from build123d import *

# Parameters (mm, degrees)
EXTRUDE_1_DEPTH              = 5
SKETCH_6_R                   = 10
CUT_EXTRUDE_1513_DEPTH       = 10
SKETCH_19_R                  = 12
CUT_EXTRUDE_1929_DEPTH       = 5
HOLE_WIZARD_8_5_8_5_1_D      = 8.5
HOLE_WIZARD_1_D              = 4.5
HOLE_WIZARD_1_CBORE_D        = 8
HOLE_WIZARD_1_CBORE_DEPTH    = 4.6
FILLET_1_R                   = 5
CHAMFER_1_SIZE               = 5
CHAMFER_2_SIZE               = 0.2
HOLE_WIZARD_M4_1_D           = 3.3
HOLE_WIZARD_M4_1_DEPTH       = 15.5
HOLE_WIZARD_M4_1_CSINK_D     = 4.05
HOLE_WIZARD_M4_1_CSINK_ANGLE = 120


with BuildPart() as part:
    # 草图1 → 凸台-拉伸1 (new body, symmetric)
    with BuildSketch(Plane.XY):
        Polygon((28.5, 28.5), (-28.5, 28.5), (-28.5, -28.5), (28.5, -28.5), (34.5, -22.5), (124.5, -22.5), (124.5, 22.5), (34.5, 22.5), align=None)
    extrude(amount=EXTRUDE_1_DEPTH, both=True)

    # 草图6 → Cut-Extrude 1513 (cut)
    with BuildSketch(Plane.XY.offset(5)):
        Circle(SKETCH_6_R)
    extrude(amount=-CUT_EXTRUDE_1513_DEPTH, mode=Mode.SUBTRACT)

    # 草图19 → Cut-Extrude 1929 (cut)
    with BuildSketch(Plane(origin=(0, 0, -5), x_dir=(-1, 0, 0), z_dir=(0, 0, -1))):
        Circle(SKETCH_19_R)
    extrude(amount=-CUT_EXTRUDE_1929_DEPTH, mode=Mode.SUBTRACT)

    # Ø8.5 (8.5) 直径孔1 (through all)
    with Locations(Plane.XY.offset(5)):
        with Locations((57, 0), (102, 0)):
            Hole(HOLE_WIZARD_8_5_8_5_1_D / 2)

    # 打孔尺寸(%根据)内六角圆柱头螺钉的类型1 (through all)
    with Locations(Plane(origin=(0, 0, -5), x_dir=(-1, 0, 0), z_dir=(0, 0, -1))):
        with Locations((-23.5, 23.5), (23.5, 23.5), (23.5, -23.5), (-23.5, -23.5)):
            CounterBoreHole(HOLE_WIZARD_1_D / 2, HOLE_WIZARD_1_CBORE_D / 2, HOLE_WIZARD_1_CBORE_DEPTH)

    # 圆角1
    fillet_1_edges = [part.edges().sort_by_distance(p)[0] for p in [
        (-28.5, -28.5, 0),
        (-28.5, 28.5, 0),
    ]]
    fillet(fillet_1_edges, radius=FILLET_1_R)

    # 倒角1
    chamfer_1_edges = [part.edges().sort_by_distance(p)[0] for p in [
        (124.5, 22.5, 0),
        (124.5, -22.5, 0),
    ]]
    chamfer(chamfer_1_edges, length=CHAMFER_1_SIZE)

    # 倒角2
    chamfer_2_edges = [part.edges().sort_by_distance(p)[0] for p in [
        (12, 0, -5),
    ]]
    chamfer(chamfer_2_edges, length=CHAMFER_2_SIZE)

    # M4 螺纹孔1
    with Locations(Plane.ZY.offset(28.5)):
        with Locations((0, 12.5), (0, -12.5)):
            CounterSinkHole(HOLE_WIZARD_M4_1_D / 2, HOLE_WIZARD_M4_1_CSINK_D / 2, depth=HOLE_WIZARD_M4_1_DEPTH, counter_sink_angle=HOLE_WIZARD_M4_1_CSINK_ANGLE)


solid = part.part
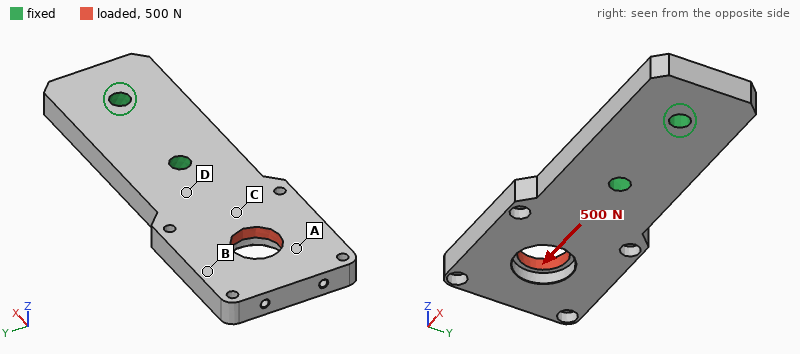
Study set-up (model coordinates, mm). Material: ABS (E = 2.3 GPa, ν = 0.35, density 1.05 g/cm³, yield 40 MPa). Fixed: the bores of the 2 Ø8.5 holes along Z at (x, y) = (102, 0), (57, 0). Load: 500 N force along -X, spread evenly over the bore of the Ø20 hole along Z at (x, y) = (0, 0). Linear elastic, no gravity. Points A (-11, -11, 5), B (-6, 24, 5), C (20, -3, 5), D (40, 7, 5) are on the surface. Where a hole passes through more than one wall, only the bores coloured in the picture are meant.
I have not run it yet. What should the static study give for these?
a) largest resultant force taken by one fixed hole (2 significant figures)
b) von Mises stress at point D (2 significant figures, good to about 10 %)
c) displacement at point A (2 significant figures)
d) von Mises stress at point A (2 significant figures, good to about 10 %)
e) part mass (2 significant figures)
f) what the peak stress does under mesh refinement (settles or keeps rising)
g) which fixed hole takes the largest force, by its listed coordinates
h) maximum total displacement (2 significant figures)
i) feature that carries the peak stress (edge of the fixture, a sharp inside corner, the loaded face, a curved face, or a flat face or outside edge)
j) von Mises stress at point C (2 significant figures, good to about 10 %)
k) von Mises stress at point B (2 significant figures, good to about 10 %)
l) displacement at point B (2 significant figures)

410 N
2.8 MPa
0.31 mm
1.7 MPa
73 g
keeps rising
(57, 0)
0.46 mm
edge of the fixture
2.4 MPa
0.86 MPa
0.27 mm
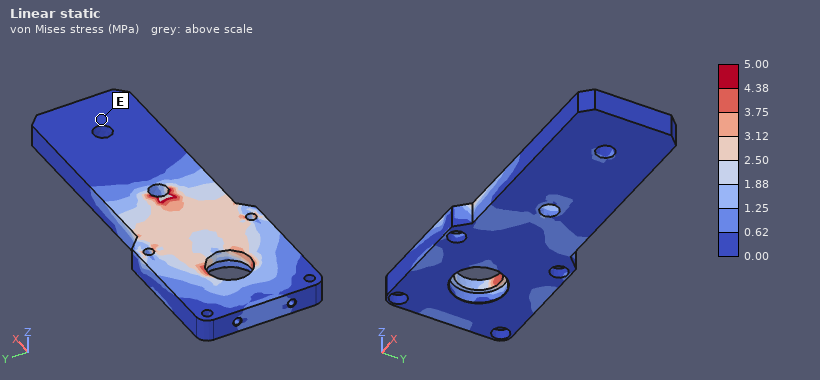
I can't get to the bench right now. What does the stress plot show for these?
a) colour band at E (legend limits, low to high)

0.00 to 0.62 MPa
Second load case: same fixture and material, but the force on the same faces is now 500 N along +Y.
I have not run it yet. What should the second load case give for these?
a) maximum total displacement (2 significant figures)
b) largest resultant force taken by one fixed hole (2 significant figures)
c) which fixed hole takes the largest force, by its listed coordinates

0.79 mm
960 N
(57, 0)
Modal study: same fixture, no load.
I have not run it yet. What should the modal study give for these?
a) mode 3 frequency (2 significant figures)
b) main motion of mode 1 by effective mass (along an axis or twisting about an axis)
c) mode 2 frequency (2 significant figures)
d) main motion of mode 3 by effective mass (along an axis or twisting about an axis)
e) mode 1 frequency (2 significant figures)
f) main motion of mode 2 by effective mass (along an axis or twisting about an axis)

880 Hz
along Z
820 Hz
along Y
320 Hz
twisting about X
